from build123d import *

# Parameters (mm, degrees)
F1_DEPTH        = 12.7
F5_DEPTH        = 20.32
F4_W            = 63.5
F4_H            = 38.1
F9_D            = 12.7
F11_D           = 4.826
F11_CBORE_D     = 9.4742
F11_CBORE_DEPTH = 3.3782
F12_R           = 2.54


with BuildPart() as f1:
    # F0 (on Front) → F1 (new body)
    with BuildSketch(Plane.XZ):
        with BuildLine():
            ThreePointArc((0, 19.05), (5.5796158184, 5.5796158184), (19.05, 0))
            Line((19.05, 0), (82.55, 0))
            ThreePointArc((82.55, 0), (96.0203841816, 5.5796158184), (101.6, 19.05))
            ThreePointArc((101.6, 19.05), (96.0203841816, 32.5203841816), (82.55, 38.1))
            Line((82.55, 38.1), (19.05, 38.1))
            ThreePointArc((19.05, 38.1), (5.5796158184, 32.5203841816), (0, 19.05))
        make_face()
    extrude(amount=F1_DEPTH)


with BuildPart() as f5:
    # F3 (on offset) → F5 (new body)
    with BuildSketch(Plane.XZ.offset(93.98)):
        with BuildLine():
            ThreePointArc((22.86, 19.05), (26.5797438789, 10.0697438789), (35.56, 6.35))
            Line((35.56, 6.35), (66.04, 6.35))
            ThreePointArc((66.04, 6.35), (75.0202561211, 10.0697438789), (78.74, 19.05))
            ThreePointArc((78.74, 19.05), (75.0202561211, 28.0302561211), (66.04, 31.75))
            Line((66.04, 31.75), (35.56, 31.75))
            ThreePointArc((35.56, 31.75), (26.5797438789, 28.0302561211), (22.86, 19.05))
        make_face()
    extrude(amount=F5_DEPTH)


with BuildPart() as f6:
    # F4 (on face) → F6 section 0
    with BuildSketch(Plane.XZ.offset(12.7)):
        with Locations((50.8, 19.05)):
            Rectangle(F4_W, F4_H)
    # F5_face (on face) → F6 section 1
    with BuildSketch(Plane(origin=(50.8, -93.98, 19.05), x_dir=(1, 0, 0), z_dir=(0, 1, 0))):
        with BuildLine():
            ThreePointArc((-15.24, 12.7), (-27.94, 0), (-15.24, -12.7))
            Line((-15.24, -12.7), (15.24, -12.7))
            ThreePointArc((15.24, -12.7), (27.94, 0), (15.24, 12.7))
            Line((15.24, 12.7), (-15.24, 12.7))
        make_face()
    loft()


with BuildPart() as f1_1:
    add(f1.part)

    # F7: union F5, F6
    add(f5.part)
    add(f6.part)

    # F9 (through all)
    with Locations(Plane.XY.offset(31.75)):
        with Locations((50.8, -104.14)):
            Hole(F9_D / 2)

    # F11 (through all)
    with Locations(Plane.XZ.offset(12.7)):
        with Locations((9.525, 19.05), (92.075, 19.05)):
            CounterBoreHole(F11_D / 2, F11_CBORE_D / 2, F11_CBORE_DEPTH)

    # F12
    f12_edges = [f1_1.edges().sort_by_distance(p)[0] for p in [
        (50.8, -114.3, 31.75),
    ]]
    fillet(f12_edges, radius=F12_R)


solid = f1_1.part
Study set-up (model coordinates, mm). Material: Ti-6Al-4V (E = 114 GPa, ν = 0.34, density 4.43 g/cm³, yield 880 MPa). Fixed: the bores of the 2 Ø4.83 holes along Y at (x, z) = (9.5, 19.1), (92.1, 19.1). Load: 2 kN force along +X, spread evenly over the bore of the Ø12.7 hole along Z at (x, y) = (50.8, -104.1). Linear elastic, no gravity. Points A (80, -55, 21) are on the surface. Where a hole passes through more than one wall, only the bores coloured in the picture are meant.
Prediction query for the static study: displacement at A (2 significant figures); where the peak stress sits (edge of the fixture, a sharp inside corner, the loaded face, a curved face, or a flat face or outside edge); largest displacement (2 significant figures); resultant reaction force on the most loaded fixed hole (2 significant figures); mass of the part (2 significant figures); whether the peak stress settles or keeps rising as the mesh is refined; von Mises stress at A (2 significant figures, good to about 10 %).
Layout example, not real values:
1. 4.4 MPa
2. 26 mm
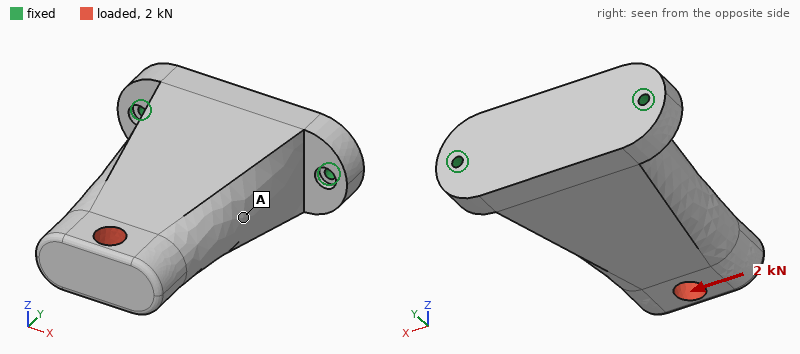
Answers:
1. 13 µm
2. edge of the fixture
3. 30 µm
4. 2.8 kN
5. 940 g
6. keeps rising
7. 6.5 MPa
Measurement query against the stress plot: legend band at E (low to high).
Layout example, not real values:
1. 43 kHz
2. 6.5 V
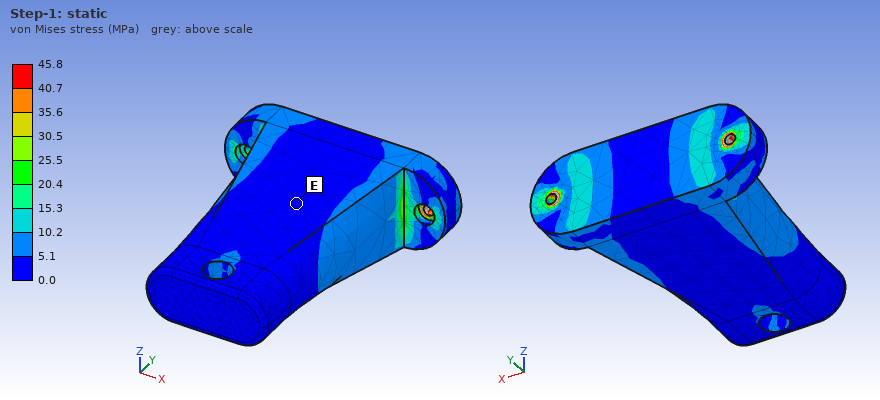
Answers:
1. 0.0 to 5.1 MPa
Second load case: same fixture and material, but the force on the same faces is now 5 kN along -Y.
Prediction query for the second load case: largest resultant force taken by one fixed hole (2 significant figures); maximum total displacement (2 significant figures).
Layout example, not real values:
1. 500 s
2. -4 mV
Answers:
1. 2.8 kN
2. 11 µm
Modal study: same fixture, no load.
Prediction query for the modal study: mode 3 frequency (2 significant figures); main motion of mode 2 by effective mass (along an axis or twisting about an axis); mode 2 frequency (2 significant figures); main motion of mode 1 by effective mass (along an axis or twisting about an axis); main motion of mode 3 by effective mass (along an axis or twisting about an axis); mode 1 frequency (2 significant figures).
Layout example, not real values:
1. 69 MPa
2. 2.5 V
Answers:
1. 4600 Hz
2. along X
3. 2800 Hz
4. along Z
5. along Y
6. 730 Hz
